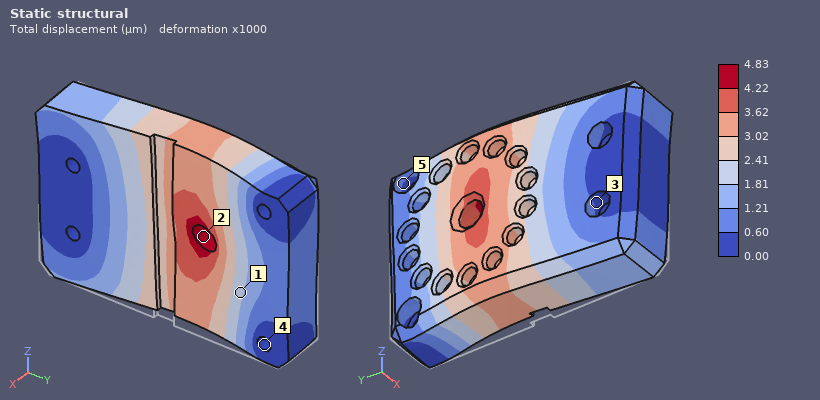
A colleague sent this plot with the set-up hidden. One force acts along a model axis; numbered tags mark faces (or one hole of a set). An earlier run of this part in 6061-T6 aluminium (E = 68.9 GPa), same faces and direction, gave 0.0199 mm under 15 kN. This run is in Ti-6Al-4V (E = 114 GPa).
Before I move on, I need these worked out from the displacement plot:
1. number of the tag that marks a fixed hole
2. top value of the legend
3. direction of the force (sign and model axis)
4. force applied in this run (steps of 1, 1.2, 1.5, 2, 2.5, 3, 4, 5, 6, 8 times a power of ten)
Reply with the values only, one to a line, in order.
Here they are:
4
4.83 µm
+Z
6 kN
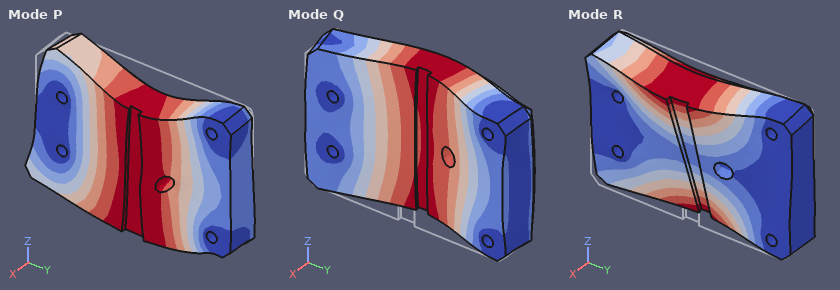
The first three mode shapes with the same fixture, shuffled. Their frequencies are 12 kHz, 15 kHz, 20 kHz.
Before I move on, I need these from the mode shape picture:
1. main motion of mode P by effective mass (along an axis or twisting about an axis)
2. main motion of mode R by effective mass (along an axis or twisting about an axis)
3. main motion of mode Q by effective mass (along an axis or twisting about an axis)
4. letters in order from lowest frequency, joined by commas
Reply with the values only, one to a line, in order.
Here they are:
along Z
twisting about Y
along X
Q, R, P
